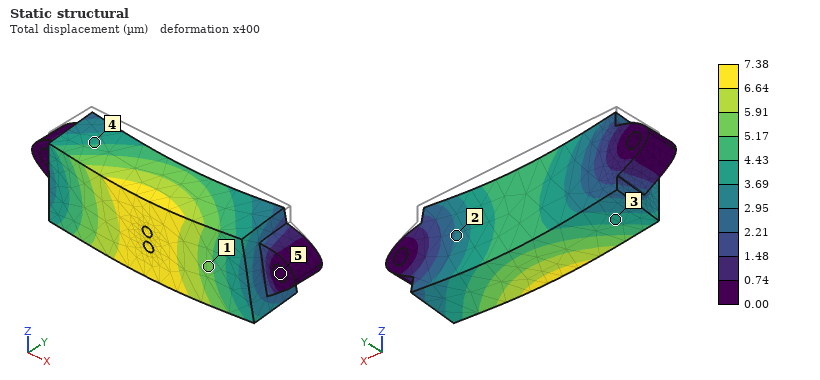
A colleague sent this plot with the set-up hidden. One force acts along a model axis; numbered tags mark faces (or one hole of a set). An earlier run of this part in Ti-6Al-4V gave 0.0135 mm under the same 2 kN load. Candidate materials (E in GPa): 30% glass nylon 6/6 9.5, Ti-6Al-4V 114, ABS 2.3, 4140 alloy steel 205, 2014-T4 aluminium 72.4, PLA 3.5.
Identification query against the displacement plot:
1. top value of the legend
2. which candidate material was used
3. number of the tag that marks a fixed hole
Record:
7.38 µm
4140 alloy steel
5
